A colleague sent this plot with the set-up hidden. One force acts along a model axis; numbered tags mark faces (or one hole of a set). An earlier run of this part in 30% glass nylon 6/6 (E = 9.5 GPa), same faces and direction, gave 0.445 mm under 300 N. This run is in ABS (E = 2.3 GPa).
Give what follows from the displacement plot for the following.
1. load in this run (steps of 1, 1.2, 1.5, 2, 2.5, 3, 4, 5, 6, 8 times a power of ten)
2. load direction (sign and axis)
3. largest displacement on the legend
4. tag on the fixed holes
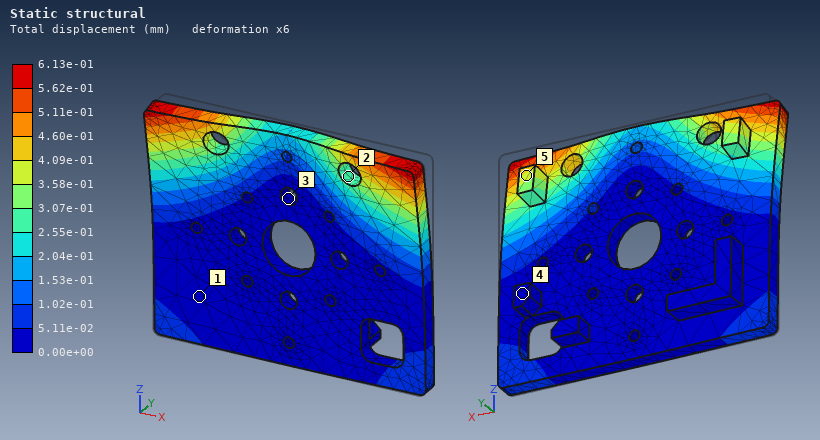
100 N
-Y
6.13e-01 mm
3
